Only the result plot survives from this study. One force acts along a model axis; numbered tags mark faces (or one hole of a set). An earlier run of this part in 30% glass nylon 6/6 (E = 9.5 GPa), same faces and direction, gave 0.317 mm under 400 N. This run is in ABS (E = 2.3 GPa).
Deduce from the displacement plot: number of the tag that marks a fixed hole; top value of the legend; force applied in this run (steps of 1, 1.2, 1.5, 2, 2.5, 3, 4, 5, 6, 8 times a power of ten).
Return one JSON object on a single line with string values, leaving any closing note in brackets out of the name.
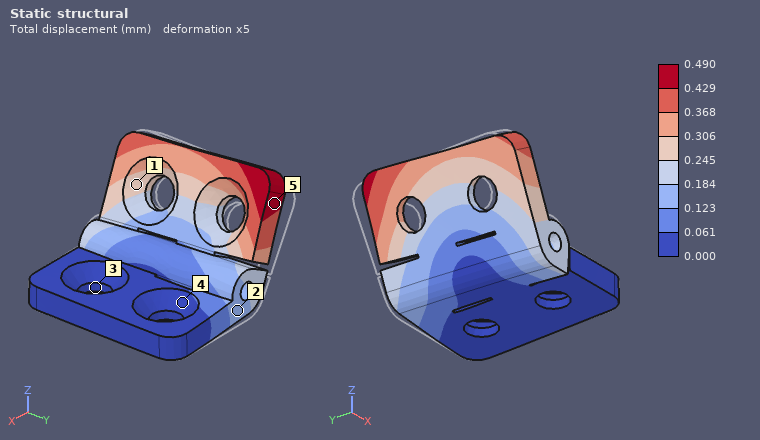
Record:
{"number of the tag that marks a fixed hole": "3", "top value of the legend": "0.490 mm", "force applied in this run": "150 N"}
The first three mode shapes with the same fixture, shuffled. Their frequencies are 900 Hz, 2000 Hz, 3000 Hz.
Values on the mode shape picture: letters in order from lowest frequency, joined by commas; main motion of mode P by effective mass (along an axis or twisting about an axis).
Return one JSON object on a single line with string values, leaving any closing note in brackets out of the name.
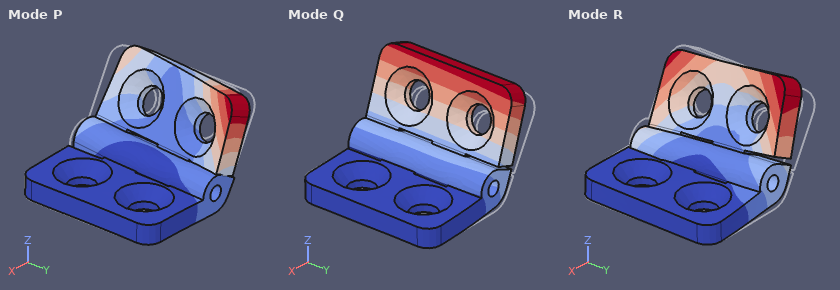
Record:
{"letters in order from lowest frequency, joined by commas": "Q, R, P", "main motion of mode P by effective mass": "along Y"}
